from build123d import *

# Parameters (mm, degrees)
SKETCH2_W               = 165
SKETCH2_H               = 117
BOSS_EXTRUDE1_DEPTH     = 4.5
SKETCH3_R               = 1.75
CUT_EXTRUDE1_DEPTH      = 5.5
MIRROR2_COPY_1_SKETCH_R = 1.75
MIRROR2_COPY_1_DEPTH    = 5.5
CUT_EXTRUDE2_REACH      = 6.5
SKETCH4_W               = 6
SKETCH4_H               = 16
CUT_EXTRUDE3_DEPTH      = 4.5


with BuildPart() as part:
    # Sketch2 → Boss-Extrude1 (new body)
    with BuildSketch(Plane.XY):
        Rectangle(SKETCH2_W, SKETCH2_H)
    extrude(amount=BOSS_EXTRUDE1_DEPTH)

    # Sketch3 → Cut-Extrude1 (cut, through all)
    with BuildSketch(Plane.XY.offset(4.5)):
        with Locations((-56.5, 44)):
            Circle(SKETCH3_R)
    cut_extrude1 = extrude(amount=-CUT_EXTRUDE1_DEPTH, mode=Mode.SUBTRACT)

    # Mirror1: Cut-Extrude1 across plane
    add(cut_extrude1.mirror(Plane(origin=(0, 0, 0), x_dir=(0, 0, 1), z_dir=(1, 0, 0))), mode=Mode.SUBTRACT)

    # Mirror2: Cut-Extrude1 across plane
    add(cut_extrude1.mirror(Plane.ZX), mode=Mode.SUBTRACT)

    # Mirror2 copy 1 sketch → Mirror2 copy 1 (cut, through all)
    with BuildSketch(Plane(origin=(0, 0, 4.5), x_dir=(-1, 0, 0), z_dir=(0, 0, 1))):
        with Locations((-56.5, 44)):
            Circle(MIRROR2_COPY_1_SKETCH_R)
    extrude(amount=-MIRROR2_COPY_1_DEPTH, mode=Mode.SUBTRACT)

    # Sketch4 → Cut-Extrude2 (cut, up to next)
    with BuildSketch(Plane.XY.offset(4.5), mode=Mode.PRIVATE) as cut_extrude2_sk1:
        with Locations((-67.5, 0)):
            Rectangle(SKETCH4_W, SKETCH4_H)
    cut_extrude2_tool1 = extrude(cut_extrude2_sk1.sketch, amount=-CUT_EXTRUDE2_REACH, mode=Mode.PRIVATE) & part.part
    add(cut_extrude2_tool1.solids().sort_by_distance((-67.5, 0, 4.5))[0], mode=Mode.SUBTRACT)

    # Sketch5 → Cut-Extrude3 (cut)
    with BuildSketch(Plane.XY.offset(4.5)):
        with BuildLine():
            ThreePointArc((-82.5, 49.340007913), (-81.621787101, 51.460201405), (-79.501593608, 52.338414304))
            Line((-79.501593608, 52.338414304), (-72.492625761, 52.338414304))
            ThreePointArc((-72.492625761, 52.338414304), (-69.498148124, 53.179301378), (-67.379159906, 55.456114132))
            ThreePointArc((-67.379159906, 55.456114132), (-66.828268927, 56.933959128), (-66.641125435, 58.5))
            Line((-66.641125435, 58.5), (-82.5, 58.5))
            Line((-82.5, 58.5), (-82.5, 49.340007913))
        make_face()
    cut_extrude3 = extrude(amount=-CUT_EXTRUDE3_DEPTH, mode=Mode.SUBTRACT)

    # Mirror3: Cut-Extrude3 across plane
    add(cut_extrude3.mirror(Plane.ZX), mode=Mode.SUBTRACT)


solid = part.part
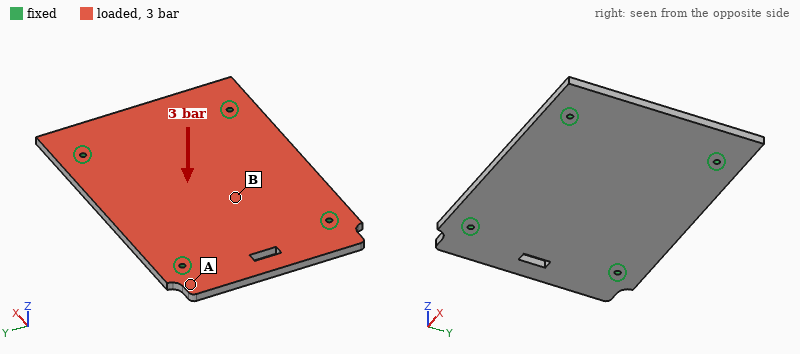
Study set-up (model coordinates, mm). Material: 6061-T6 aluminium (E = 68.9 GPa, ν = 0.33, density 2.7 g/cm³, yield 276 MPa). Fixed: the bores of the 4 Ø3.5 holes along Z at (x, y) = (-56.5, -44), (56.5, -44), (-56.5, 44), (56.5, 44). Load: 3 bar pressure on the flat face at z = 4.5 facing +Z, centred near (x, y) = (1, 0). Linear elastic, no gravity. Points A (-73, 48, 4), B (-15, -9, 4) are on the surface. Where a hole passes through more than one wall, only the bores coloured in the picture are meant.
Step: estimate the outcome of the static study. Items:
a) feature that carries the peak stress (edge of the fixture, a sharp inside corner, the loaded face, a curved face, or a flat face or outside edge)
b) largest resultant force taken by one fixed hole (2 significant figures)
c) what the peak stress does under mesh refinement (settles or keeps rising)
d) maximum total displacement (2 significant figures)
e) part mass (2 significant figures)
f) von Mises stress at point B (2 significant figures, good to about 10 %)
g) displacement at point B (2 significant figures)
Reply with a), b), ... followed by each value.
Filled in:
a) edge of the fixture
b) 1.4 kN
c) keeps rising
d) 0.44 mm
e) 230 g
f) 45 MPa
g) 0.41 mm
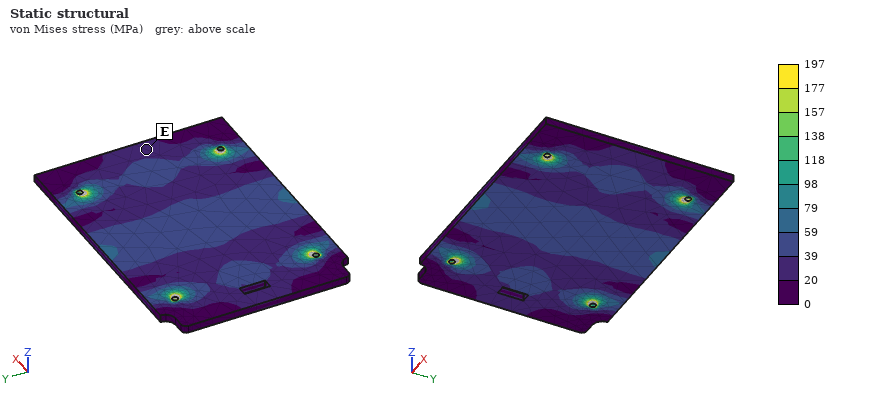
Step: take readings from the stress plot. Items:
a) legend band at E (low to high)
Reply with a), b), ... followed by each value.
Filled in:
a) 20 to 39 MPa
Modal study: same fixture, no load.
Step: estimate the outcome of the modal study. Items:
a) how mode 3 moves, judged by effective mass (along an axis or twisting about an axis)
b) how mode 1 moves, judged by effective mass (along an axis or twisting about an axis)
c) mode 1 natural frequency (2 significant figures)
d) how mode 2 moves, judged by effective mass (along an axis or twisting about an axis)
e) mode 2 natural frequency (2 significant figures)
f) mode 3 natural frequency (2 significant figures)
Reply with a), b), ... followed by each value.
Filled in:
a) along Z
b) along Z
c) 1400 Hz
d) twisting about X
e) 2000 Hz
f) 2300 Hz
